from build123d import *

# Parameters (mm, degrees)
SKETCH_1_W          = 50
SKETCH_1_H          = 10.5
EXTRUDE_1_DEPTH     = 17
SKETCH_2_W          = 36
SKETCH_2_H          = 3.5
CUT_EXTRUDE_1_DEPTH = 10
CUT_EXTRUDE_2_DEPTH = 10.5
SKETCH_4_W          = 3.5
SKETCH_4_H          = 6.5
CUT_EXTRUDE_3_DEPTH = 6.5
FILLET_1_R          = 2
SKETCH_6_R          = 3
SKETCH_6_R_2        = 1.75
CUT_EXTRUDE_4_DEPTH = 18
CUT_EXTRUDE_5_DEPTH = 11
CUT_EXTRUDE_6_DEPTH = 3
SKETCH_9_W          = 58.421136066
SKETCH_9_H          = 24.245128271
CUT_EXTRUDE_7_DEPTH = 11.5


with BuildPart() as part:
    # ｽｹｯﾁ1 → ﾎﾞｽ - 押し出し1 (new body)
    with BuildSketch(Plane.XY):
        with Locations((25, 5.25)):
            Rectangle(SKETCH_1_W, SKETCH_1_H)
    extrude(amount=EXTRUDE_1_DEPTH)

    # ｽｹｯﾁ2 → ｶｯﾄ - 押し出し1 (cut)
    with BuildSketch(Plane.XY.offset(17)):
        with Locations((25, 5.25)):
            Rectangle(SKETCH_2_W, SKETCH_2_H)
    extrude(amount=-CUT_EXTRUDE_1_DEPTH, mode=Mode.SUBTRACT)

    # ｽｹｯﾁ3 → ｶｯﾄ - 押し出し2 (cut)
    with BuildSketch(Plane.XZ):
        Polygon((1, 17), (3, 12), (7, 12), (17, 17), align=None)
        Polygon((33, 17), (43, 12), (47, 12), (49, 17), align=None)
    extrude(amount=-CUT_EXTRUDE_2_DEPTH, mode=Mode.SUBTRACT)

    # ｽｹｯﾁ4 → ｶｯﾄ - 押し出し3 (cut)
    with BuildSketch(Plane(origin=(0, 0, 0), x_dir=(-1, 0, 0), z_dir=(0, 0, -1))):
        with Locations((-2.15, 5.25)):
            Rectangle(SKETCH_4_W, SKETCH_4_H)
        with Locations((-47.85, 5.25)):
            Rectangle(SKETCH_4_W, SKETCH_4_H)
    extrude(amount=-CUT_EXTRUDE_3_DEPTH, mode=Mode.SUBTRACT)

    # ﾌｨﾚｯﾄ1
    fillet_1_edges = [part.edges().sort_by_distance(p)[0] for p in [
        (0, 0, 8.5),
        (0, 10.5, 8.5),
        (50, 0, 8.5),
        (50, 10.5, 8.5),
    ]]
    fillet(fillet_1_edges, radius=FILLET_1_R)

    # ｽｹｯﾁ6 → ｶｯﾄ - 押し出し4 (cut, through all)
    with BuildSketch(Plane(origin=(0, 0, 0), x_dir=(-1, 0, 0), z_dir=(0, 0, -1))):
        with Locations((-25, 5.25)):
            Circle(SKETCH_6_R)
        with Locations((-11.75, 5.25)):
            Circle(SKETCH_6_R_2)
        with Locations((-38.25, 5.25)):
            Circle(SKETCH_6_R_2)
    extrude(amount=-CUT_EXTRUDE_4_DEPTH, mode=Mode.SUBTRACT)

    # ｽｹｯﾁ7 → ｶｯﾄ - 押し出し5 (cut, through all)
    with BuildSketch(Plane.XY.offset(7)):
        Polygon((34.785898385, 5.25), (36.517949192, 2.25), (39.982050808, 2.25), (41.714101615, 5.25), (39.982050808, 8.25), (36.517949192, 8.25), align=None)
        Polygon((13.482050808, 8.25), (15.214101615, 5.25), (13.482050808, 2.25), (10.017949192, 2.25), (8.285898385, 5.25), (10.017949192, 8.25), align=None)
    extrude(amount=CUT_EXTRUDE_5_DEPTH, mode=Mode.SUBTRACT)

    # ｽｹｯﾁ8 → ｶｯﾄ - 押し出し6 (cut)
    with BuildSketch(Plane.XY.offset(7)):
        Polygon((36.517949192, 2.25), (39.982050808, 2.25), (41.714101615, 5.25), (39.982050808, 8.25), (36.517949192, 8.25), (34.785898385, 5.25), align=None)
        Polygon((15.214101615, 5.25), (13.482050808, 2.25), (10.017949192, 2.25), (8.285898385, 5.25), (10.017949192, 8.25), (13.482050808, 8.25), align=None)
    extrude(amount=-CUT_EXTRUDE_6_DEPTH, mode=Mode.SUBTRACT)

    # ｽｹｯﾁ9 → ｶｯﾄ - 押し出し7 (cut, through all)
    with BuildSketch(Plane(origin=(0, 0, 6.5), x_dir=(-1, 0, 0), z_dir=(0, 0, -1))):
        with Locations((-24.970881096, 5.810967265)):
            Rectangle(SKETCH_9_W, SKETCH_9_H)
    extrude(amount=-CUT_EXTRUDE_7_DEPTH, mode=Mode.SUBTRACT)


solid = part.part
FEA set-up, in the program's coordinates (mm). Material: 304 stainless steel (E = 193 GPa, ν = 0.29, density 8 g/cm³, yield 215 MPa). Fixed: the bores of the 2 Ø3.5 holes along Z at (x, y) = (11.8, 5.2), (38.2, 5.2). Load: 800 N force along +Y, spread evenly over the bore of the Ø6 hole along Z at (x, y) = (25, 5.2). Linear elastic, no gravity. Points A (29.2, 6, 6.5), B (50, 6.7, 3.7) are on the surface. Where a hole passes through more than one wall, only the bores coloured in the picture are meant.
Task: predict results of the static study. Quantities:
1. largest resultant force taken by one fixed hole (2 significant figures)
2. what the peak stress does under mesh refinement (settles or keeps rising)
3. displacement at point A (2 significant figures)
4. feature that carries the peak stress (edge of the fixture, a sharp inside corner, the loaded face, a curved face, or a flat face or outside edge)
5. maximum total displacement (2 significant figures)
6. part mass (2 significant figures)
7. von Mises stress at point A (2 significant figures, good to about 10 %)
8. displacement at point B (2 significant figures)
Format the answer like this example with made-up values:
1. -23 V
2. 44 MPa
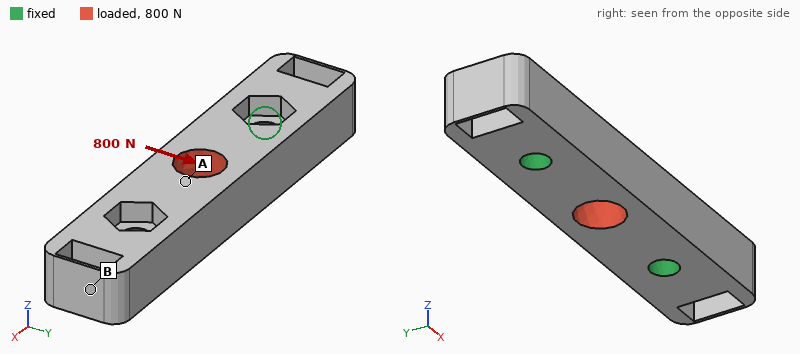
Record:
1. 400 N
2. keeps rising
3. 2.2 µm
4. edge of the fixture
5. 2.8 µm
6. 21 g
7. 17 MPa
8. 1.1 µm
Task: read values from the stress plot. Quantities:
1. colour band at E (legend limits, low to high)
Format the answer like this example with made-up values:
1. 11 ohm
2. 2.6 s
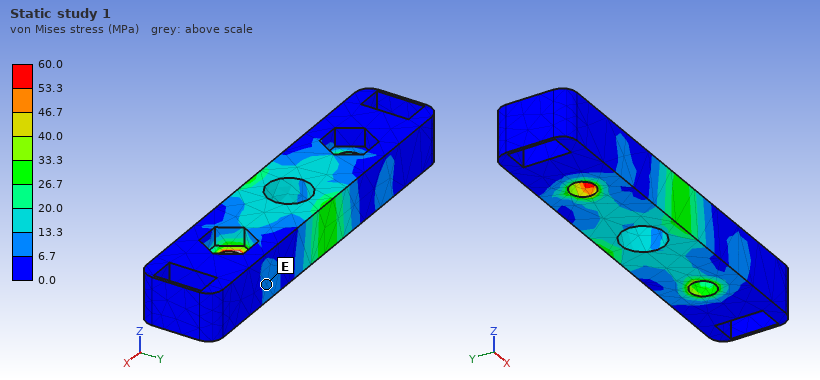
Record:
1. 6.7 to 13.3 MPa
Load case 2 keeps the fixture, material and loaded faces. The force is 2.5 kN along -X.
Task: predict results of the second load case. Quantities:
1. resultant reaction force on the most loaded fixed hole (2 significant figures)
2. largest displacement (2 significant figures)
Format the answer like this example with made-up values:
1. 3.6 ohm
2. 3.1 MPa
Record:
1. 1.3 kN
2. 1.7 µm
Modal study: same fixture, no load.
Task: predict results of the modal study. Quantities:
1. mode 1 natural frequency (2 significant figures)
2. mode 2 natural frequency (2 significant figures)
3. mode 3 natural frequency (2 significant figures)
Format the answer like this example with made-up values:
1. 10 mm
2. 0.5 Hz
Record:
1. 27 kHz
2. 31 kHz
3. 31 kHz
